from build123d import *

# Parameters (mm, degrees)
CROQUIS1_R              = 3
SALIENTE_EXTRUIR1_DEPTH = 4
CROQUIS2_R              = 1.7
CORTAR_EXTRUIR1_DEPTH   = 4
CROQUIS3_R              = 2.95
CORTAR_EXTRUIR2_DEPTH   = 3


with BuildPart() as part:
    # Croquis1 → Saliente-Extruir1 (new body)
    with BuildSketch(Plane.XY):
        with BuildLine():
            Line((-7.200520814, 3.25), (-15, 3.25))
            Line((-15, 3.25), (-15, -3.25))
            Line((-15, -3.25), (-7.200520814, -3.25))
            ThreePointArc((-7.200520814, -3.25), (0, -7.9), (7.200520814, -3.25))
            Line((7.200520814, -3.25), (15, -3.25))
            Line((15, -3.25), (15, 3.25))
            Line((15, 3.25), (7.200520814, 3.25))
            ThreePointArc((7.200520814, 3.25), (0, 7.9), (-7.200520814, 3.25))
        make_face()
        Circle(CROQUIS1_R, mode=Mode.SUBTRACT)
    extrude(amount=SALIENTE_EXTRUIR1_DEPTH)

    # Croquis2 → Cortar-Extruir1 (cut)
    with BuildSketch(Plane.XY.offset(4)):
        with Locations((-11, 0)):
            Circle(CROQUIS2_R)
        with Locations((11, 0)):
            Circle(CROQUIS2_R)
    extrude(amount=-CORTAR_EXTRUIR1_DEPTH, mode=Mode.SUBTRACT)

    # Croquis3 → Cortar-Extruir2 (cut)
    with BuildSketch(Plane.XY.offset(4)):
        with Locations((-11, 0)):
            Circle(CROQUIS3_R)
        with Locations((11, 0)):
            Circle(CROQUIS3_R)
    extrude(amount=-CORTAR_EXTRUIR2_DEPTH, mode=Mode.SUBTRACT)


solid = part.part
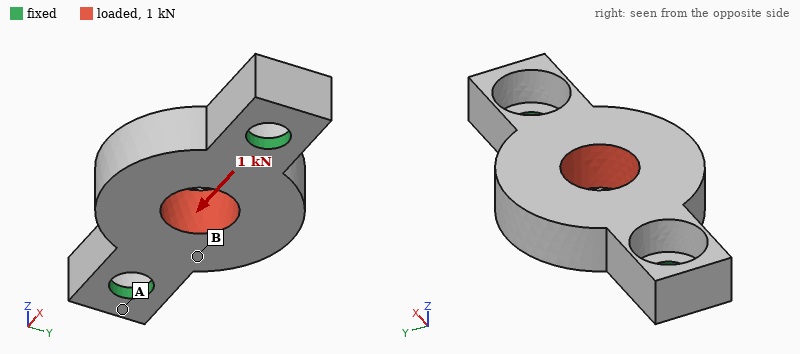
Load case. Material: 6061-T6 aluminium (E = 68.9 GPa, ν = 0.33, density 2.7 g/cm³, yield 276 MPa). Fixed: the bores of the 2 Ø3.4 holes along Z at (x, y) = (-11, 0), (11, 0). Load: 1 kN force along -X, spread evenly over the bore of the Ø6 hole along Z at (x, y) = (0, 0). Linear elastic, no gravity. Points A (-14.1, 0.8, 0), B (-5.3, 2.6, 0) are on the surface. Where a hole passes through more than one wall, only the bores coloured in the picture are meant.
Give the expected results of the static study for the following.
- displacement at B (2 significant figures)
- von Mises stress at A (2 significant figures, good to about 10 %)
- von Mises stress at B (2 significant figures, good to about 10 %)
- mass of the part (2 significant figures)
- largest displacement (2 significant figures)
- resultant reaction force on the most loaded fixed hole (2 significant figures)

3.8 µm
16 MPa
34 MPa
2.3 g
5.4 µm
500 N
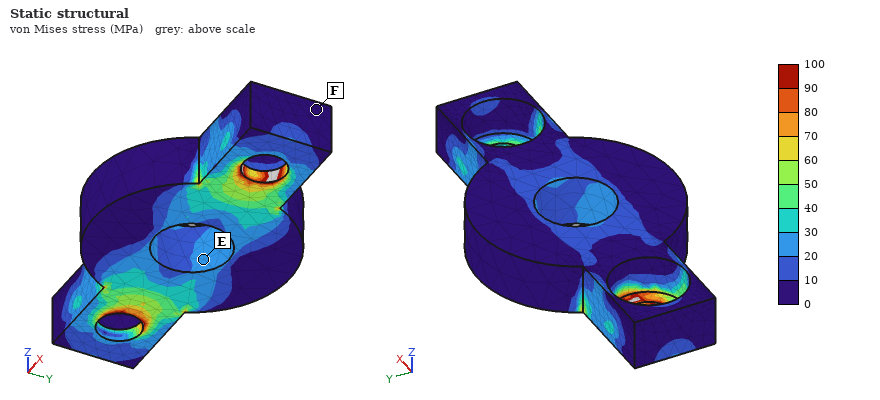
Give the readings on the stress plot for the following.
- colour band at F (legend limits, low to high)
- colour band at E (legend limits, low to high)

0 to 10 MPa
20 to 30 MPa
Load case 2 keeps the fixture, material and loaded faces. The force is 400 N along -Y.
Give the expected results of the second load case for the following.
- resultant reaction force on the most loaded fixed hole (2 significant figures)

200 N
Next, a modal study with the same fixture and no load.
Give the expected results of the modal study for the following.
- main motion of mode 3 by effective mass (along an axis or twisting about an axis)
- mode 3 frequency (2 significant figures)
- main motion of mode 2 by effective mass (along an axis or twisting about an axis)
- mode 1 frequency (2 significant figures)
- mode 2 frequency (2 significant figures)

along Y
37 kHz
along Z
13 kHz
21 kHz
